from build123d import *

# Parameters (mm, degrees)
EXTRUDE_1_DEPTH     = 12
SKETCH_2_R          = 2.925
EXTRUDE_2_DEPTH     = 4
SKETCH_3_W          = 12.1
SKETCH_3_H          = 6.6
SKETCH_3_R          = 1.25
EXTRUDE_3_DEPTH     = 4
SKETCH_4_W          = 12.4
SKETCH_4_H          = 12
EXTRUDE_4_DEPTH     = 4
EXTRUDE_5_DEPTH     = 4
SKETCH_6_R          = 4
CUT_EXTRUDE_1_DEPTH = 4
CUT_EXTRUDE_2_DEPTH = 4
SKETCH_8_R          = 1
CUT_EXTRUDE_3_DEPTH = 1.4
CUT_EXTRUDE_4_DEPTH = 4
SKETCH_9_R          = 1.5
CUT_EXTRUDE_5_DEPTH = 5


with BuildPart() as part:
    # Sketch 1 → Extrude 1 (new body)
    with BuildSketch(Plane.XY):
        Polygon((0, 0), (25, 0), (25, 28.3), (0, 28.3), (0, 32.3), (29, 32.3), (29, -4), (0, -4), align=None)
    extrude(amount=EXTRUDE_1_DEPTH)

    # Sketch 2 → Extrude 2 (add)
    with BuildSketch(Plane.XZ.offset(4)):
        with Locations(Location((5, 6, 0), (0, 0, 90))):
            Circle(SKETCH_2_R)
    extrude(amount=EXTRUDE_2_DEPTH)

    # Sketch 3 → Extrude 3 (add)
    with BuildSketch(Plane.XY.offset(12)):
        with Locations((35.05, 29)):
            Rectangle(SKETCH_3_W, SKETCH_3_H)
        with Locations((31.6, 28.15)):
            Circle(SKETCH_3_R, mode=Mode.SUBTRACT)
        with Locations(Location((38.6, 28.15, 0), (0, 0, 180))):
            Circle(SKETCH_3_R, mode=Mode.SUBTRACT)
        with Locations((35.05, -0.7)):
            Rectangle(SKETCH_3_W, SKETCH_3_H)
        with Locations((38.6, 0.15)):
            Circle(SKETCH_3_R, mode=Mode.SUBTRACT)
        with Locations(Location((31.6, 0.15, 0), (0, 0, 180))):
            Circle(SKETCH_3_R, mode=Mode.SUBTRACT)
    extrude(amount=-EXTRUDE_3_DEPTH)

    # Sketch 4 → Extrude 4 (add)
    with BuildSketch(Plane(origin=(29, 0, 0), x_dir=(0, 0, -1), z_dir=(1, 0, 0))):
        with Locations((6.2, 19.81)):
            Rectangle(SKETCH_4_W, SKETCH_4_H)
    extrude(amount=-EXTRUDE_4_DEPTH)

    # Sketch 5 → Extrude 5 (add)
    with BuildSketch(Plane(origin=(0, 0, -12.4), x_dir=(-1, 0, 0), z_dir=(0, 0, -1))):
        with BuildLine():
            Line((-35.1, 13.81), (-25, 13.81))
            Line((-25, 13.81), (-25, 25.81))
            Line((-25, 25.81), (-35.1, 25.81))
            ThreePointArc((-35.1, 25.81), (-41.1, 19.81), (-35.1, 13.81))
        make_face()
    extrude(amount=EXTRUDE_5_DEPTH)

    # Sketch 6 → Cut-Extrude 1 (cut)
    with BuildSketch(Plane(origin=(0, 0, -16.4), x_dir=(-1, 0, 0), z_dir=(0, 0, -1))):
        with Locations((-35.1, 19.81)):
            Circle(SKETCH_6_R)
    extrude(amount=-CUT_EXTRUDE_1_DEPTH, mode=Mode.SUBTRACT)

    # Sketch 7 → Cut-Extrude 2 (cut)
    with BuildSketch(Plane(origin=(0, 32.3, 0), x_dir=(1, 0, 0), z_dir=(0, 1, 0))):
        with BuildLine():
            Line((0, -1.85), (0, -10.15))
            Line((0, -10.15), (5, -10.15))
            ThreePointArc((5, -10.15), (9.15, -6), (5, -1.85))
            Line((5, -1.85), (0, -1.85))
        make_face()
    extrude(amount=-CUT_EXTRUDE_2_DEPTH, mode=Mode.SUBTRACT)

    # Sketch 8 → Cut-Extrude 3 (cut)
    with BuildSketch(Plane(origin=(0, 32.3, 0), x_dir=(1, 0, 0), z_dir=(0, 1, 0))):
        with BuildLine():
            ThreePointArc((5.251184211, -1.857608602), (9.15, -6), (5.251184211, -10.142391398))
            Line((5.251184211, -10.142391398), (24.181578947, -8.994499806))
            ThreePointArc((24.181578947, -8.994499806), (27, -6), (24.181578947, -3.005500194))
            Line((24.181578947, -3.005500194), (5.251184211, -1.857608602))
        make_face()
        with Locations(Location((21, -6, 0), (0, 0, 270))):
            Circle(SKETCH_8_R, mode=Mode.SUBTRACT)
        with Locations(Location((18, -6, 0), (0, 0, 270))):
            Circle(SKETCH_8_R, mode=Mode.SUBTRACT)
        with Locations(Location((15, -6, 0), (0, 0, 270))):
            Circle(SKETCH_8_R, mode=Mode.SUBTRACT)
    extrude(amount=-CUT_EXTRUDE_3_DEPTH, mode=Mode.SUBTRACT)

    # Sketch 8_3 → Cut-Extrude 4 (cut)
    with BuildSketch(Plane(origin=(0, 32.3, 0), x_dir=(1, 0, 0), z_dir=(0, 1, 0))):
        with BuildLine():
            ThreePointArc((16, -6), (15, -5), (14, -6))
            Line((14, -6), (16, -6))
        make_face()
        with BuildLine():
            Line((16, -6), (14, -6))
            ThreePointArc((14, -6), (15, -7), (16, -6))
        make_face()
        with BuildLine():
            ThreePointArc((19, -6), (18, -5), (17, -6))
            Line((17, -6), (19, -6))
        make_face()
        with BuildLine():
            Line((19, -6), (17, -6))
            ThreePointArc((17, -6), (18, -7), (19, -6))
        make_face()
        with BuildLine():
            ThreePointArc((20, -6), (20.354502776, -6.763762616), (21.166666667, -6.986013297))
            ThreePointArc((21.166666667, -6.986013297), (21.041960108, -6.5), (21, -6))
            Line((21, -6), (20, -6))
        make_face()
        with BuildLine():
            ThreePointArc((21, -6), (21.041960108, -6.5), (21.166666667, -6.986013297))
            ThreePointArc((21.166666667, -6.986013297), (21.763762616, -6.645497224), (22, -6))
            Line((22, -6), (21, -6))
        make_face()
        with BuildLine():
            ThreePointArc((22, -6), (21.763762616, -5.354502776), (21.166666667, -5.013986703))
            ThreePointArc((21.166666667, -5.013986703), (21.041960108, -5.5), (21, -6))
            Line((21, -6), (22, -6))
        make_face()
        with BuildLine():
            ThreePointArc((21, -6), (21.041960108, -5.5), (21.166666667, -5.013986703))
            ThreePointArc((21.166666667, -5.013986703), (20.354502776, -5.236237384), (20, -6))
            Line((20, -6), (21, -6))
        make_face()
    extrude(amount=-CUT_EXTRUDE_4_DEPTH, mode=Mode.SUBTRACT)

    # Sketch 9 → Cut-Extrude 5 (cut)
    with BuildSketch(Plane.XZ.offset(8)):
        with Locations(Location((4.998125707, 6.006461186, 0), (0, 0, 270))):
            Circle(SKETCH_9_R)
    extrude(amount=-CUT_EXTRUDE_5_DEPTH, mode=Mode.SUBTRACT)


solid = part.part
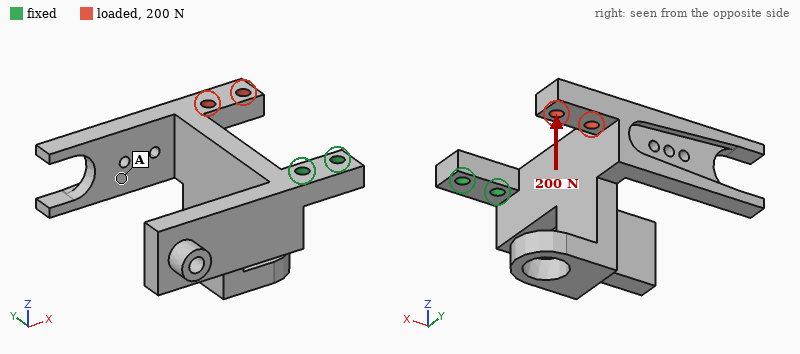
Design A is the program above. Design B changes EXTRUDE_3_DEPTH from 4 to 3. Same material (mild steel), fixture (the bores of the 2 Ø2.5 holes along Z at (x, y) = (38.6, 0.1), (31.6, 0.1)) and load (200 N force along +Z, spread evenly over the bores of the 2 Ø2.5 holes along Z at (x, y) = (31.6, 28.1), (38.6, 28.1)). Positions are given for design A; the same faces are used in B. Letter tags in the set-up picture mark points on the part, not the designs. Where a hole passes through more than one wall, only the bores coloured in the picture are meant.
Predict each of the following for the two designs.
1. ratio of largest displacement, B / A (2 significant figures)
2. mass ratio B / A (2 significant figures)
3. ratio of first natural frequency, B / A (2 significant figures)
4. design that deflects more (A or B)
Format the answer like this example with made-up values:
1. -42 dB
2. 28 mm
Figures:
1. 1.5
2. 0.97
3. 0.89
4. B
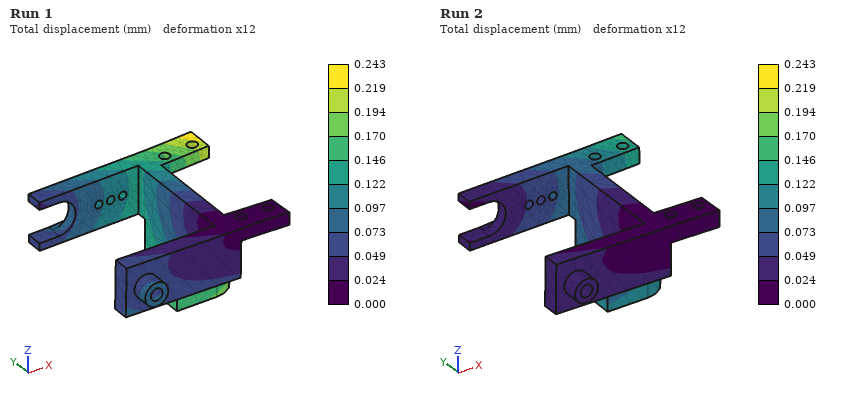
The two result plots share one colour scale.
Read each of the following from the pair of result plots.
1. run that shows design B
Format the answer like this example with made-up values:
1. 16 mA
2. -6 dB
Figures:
1. Run 1
